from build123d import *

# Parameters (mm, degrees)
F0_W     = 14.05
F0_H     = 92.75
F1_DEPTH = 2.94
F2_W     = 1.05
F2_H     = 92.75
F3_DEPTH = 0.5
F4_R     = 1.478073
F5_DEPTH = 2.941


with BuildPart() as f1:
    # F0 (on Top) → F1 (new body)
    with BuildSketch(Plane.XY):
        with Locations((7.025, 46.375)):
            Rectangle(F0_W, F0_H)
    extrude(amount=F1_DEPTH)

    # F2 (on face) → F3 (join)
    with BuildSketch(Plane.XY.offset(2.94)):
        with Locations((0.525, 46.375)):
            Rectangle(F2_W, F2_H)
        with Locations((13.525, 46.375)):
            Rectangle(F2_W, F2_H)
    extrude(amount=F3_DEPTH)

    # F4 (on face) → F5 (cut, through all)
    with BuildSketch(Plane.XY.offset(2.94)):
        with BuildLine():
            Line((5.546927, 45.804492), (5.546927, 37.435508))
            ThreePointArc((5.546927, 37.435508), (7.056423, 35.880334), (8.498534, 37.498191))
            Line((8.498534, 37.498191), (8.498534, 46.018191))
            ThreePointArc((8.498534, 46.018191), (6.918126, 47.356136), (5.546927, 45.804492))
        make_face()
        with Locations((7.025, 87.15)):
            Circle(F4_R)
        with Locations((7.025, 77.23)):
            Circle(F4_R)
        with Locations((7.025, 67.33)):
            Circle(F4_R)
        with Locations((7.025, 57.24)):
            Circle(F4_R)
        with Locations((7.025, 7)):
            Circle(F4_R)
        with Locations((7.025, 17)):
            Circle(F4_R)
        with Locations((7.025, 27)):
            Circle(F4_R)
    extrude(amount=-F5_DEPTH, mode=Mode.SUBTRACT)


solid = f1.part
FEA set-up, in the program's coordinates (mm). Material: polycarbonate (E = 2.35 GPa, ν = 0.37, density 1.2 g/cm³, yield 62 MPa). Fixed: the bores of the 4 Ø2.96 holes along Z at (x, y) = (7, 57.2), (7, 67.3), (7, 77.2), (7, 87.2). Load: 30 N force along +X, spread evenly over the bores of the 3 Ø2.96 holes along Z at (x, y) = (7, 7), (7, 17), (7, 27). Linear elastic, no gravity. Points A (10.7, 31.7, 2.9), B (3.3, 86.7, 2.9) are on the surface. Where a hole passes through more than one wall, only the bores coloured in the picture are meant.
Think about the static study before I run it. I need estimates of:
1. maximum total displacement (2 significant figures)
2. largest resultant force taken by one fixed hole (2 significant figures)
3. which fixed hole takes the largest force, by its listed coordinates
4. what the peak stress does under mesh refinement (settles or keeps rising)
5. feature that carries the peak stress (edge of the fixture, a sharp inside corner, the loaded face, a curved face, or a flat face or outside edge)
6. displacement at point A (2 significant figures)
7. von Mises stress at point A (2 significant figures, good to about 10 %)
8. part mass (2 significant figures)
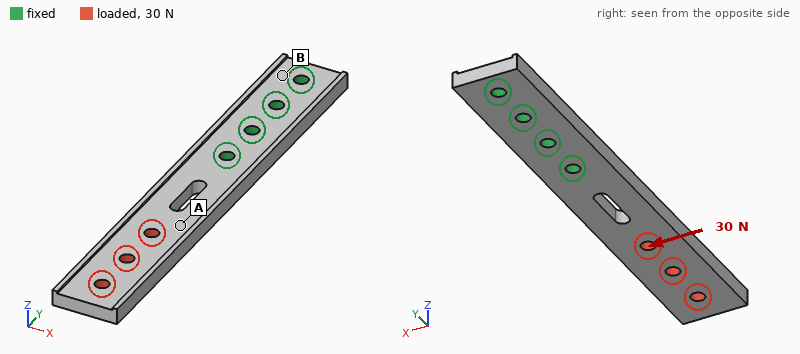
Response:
0.97 mm
96 N
(7, 57.2)
keeps rising
edge of the fixture
0.36 mm
2.9 MPa
4.4 g
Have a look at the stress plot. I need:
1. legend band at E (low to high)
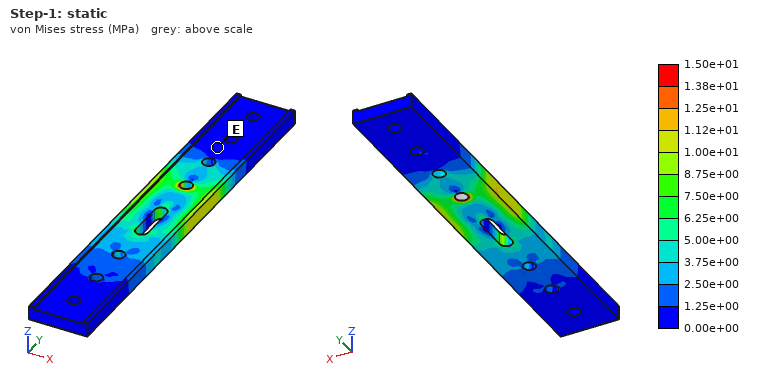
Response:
0.00e+00 to 1.25e+00 MPa
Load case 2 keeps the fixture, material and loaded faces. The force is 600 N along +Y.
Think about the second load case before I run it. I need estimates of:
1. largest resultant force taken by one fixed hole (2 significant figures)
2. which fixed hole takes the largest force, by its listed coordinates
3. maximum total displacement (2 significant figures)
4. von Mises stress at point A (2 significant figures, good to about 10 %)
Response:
470 N
(7, 57.2)
0.64 mm
14 MPa
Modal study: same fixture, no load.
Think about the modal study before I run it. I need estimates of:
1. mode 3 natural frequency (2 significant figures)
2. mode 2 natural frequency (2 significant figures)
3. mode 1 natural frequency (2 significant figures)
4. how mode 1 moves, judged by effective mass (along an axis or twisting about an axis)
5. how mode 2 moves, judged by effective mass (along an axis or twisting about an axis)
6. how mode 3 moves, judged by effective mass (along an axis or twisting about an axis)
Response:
1300 Hz
790 Hz
210 Hz
along Z
along X
twisting about Y
